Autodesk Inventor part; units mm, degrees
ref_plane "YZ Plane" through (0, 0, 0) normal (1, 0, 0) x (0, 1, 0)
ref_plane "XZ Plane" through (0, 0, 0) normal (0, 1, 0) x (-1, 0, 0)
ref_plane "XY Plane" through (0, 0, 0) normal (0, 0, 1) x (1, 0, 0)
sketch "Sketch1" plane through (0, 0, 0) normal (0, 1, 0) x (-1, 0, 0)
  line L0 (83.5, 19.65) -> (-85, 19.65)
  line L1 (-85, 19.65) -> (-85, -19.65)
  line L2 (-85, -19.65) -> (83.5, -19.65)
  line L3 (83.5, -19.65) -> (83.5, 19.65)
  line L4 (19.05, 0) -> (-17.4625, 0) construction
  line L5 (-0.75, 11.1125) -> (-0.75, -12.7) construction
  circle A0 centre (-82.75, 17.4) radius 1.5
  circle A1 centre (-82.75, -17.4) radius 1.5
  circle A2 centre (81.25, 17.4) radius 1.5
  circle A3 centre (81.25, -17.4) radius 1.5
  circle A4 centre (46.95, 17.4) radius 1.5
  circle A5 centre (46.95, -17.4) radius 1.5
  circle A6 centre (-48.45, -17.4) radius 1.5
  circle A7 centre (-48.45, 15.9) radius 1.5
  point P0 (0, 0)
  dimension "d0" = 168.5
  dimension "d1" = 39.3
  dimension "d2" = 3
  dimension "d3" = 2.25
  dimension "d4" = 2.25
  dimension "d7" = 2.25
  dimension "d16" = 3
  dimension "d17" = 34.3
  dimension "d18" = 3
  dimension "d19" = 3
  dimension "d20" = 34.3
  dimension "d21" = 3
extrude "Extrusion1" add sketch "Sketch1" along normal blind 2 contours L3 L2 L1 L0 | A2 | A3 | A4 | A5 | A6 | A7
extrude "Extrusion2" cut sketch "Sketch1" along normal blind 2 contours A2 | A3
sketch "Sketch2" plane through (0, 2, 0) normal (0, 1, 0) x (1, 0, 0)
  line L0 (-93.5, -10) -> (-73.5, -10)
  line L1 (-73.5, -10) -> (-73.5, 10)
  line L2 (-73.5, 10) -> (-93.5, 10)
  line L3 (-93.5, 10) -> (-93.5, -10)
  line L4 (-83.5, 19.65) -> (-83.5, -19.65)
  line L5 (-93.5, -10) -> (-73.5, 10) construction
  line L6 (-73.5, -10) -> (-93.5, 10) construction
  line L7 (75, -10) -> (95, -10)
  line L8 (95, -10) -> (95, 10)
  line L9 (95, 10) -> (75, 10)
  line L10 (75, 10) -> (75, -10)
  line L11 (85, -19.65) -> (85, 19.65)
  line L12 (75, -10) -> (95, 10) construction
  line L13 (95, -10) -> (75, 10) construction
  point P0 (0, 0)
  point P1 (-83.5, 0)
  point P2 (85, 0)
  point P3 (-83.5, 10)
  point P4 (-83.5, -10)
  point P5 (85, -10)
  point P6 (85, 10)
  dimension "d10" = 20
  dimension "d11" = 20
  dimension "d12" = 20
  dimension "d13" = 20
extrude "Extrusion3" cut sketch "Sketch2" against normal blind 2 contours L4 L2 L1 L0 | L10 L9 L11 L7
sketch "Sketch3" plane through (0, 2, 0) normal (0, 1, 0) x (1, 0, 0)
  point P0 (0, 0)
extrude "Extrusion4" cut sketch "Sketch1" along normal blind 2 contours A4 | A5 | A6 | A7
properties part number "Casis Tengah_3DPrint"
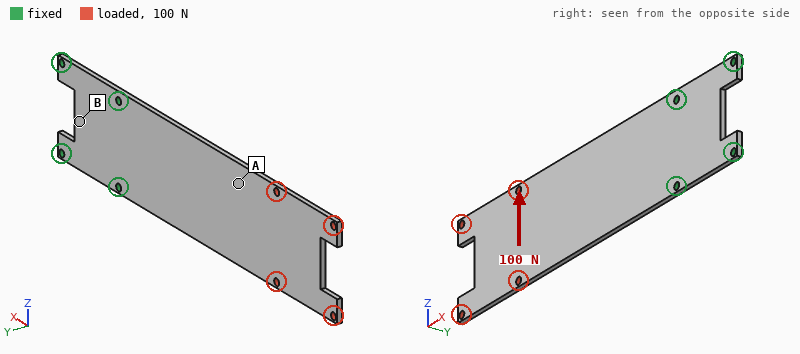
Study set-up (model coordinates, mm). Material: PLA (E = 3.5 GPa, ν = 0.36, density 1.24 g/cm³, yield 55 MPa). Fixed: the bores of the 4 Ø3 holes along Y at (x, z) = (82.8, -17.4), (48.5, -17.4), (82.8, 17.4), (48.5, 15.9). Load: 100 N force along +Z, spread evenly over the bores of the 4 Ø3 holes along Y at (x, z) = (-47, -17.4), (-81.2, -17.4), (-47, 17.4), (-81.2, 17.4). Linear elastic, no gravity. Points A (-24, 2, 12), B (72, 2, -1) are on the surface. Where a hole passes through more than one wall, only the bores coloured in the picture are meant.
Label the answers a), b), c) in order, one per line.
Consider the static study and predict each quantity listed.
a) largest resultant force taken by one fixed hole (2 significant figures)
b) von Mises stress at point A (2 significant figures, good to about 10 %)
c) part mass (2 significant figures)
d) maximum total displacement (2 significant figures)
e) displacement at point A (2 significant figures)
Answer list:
a) 330 N
b) 5.2 MPa
c) 15 g
d) 2.0 mm
e) 0.77 mm
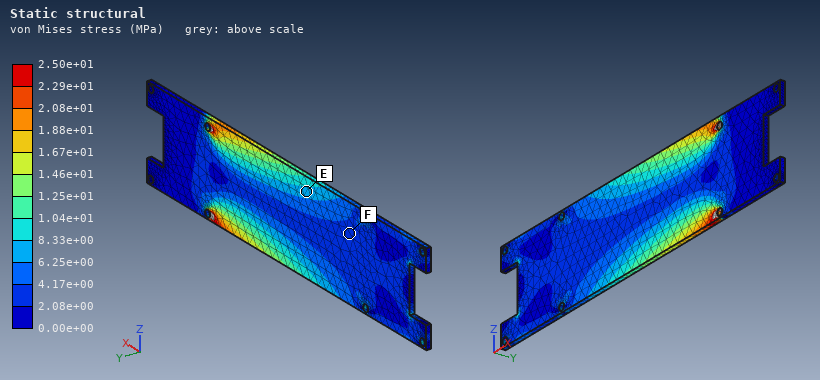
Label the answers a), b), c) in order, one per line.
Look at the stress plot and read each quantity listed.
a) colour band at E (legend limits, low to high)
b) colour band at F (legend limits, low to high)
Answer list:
a) 6.25e+00 to 8.33e+00 MPa
b) 2.08e+00 to 4.17e+00 MPa
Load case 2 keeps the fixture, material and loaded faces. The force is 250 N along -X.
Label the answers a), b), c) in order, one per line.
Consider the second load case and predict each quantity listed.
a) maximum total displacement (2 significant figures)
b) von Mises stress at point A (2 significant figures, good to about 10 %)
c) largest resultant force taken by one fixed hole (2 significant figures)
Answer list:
a) 0.17 mm
b) 3.2 MPa
c) 110 N
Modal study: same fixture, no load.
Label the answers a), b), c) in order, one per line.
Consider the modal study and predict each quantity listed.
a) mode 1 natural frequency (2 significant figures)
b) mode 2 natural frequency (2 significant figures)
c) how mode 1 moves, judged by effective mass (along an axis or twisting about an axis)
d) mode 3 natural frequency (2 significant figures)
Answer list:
a) 33 Hz
b) 210 Hz
c) along Y
d) 210 Hz
